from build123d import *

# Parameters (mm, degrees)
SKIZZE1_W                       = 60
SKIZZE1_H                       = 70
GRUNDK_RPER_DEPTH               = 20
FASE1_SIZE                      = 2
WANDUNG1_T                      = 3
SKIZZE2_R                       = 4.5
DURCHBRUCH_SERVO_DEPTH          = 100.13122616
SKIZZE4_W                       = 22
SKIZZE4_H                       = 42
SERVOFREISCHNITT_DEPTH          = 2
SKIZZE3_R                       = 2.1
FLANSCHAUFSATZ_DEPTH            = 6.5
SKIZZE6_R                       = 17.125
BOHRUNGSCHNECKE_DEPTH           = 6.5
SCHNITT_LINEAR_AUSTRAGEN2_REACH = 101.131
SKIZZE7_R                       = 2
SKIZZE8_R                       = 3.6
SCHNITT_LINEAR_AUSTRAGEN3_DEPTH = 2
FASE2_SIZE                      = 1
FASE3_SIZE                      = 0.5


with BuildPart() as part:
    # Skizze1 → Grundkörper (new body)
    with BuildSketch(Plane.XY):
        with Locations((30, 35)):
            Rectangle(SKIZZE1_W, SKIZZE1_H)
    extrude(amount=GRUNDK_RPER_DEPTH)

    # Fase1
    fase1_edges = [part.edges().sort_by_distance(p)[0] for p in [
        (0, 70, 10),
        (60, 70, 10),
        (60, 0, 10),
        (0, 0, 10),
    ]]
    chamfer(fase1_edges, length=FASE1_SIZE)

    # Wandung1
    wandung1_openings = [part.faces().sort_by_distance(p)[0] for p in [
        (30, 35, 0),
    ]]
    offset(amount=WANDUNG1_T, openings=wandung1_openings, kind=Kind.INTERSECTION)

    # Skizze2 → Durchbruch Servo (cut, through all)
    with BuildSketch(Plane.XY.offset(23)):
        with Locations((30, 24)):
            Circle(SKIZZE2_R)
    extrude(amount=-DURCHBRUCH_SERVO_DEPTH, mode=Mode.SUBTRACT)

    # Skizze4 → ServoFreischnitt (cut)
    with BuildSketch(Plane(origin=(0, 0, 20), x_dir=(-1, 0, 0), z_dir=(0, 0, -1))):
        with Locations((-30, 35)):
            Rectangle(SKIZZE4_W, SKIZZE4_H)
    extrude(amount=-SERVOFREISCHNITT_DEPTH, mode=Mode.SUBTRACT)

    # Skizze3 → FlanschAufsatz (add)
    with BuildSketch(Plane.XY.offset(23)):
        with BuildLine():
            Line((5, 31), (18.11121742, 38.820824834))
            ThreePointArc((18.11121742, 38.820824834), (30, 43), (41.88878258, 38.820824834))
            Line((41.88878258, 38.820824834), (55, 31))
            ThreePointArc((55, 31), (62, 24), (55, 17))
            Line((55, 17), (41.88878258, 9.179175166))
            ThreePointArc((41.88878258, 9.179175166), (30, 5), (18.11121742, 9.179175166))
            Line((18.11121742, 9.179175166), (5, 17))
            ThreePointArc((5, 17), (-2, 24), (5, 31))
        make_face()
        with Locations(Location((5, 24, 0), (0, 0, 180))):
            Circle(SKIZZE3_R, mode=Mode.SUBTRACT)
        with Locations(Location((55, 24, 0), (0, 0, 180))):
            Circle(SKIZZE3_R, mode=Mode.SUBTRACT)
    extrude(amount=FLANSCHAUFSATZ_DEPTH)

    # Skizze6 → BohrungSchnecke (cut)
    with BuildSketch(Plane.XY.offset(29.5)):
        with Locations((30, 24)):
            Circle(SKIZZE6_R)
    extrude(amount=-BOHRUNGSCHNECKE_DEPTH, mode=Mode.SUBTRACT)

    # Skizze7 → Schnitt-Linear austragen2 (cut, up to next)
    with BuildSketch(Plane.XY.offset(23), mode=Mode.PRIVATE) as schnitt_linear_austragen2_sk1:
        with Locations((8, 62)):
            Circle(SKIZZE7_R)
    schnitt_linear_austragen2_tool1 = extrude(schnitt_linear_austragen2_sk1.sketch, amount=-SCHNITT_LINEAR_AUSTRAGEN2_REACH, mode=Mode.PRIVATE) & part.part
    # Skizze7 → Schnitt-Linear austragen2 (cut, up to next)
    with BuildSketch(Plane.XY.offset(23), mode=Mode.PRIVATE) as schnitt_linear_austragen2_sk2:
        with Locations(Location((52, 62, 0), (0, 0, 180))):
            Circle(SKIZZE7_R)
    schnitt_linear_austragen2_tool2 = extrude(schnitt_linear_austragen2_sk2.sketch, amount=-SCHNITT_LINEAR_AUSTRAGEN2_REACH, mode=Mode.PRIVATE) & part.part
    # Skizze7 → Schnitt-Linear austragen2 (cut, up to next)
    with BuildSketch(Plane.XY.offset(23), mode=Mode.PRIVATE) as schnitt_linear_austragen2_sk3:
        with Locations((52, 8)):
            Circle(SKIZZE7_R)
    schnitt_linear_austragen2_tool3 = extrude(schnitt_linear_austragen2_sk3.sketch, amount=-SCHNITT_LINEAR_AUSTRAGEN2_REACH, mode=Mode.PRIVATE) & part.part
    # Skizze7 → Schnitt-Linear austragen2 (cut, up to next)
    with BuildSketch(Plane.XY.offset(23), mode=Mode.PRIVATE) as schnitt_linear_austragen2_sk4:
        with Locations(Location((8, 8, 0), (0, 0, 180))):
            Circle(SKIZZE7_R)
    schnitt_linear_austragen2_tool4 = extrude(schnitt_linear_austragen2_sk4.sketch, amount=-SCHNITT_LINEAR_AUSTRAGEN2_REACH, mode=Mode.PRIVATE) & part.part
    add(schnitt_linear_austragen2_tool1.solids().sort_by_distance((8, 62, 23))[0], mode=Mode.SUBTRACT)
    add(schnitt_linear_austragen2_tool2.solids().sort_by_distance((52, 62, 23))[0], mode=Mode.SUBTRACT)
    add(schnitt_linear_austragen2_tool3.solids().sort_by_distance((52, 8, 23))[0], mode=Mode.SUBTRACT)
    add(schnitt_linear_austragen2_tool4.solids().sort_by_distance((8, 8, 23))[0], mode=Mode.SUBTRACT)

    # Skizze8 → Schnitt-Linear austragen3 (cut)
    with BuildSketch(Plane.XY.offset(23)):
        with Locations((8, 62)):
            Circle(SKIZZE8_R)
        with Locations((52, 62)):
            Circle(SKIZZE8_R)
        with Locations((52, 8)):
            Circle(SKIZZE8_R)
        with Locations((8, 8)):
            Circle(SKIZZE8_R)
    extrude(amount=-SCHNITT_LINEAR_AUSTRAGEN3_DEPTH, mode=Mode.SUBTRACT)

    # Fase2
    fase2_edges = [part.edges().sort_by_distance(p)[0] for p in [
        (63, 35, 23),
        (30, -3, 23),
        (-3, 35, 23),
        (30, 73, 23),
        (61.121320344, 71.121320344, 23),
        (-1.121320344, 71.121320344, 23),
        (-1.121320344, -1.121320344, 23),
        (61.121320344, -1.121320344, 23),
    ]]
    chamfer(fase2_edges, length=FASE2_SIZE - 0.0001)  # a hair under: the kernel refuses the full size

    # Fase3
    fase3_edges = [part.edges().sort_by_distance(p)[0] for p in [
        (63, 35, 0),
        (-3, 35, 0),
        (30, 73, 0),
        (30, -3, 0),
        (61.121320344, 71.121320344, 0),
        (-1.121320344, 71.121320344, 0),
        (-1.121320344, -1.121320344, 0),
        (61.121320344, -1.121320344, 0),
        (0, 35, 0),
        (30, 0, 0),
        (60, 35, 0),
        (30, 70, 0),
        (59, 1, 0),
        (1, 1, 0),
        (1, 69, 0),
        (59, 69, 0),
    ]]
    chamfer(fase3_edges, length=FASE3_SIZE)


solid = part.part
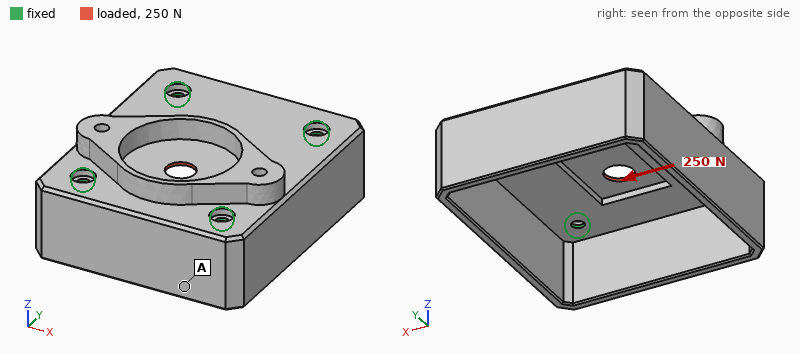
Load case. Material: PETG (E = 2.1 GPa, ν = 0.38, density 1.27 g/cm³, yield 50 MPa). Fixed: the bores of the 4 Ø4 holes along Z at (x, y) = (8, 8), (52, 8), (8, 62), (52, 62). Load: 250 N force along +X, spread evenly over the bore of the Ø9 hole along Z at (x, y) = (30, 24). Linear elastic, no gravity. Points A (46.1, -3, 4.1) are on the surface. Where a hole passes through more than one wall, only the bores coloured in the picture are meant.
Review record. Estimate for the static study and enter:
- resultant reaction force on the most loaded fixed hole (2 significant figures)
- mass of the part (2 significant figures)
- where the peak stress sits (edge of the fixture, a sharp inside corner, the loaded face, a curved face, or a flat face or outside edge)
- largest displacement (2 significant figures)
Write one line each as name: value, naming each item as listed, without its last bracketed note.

resultant reaction force on the most loaded fixed hole: 88 N
mass of the part: 41 g
where the peak stress sits: the loaded face
largest displacement: 68 µm
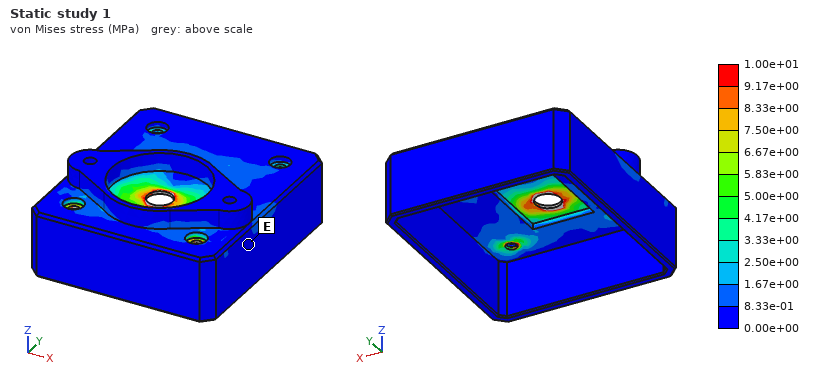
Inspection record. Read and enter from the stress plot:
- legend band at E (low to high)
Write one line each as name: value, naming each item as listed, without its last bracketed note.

legend band at E: 0.00e+00 to 8.33e-01 MPa
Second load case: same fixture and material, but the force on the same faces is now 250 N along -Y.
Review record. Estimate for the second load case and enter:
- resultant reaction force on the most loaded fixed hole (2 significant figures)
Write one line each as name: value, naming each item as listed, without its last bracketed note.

resultant reaction force on the most loaded fixed hole: 76 N
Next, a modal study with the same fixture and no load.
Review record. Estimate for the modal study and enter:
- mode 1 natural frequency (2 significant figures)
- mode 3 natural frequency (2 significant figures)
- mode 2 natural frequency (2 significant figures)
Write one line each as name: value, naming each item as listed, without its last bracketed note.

mode 1 natural frequency: 1200 Hz
mode 3 natural frequency: 1300 Hz
mode 2 natural frequency: 1200 Hz
